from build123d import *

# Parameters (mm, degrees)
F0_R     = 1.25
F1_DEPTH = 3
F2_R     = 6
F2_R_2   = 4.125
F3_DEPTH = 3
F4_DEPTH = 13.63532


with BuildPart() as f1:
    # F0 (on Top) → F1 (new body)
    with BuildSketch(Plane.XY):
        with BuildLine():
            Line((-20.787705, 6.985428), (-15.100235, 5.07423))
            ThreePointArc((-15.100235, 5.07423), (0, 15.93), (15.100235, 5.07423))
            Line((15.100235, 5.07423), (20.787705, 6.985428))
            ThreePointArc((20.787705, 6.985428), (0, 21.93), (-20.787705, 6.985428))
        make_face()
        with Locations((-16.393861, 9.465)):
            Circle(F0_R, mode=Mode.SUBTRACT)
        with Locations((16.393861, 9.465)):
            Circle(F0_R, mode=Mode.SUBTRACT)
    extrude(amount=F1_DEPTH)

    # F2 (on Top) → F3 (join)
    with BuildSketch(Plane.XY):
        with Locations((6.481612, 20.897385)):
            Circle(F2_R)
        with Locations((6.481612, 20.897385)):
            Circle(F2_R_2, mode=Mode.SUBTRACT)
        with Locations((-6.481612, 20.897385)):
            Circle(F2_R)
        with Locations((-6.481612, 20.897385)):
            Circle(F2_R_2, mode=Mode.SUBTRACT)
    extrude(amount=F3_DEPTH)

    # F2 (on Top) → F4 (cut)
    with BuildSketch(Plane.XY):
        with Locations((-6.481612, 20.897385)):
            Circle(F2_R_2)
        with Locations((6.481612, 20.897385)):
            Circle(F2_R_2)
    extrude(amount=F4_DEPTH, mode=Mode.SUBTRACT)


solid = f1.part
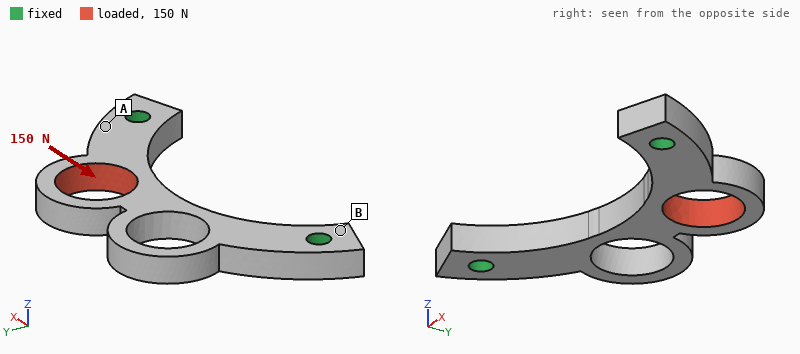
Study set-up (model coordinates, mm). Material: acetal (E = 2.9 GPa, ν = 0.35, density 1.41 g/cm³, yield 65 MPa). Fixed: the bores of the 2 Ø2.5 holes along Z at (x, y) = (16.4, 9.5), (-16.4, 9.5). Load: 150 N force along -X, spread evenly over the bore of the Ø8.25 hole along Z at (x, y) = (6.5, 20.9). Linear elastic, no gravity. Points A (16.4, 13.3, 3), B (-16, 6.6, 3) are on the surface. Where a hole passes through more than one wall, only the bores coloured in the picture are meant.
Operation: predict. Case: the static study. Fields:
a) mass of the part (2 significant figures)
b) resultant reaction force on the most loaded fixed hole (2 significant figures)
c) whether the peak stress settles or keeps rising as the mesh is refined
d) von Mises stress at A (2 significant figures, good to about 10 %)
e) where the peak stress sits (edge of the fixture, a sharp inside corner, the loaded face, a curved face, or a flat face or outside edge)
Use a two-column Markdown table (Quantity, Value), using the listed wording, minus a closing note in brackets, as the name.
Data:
| Quantity | Value |
|---|---|
| mass of the part | 1.2 g |
| resultant reaction force on the most loaded fixed hole | 88 N |
| whether the peak stress settles or keeps rising as the mesh is refined | keeps rising |
| von Mises stress at A | 9.2 MPa |
| where the peak stress sits | a sharp inside corner |
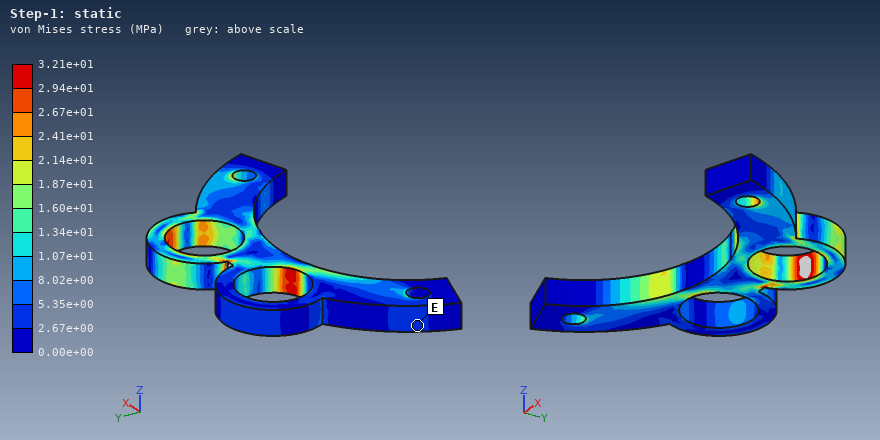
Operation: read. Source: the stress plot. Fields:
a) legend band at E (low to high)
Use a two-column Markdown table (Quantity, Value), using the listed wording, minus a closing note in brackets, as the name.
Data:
| Quantity | Value |
|---|---|
| legend band at E | 2.67e+00 to 5.35e+00 MPa |
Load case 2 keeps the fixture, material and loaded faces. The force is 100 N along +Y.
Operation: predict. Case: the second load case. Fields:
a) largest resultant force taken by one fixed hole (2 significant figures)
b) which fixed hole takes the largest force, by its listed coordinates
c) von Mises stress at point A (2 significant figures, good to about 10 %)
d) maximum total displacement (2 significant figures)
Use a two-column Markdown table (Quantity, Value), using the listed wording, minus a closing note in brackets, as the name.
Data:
| Quantity | Value |
|---|---|
| largest resultant force taken by one fixed hole | 90 N |
| which fixed hole takes the largest force, by its listed coordinates | (16.4, 9.5) |
| von Mises stress at point A | 1.9 MPa |
| maximum total displacement | 0.11 mm |
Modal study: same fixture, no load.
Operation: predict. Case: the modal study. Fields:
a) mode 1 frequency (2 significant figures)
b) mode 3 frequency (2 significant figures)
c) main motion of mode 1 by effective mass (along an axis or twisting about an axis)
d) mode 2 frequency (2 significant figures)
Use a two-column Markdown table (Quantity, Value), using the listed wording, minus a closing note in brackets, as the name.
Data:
| Quantity | Value |
|---|---|
| mode 1 frequency | 1800 Hz |
| mode 3 frequency | 5500 Hz |
| main motion of mode 1 by effective mass | along Z |
| mode 2 frequency | 4000 Hz |
